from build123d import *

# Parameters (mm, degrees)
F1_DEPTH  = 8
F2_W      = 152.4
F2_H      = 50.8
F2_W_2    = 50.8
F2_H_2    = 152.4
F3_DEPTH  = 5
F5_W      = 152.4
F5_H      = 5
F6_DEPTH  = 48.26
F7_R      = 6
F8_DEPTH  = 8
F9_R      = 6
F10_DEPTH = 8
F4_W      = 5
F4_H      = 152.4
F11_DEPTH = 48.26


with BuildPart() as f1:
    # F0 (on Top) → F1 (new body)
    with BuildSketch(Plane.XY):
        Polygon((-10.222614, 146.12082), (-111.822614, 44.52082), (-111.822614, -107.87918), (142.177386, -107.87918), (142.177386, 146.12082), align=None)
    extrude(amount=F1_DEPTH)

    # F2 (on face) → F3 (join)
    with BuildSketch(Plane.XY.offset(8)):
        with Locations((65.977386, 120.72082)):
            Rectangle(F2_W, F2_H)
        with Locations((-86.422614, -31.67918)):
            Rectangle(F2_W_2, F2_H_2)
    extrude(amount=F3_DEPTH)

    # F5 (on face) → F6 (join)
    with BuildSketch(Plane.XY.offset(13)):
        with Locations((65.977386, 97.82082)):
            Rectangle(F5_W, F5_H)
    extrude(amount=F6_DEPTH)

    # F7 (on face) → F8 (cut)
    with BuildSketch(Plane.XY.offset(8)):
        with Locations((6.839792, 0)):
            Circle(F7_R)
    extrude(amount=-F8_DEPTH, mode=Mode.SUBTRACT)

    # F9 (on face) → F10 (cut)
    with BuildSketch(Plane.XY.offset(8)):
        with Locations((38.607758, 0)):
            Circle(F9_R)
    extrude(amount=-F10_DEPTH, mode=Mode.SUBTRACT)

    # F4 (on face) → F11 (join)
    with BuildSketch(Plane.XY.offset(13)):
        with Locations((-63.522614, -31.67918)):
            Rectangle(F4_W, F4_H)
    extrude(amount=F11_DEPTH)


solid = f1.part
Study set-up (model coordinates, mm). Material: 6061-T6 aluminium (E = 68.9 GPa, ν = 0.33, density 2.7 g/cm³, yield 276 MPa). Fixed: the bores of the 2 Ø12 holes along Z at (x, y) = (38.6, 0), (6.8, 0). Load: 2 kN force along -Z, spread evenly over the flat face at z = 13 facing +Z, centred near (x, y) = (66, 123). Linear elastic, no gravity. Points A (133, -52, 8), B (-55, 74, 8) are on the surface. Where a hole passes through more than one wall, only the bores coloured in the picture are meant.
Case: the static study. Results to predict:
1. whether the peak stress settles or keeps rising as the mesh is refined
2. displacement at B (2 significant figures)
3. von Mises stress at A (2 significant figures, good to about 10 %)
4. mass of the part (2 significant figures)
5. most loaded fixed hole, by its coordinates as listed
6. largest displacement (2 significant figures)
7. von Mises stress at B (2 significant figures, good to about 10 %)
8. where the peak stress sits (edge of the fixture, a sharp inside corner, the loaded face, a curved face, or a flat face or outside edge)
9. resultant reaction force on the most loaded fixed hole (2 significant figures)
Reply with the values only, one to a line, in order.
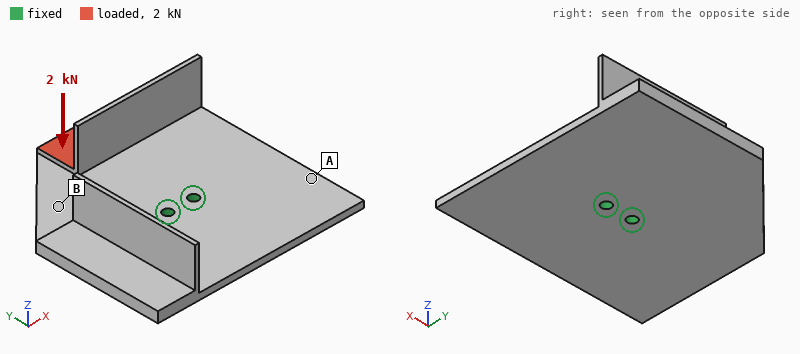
keeps rising
0.58 mm
19 MPa
1.7 kg
(38.6, 0)
3.8 mm
56 MPa
edge of the fixture
2.4 kN
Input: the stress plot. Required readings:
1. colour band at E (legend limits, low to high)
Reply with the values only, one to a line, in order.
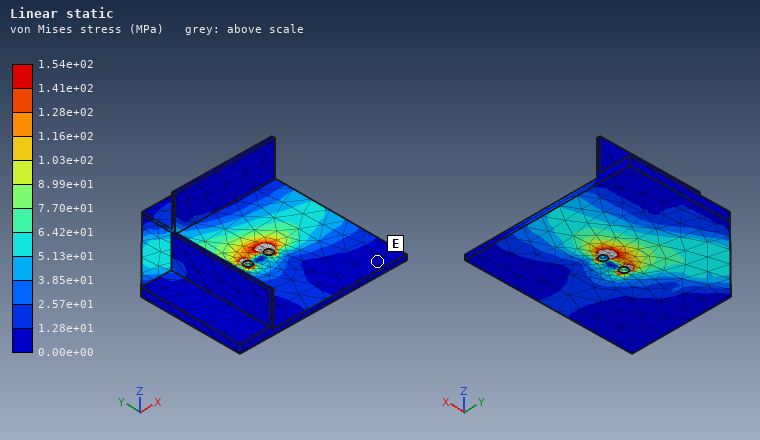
0.00e+00 to 1.28e+01 MPa
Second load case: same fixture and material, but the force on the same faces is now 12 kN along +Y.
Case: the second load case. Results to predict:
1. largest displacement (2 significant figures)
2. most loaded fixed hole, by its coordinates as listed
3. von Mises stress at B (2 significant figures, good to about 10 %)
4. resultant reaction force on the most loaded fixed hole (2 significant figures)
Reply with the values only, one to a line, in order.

2.0 mm
(38.6, 0)
38 MPa
19 kN
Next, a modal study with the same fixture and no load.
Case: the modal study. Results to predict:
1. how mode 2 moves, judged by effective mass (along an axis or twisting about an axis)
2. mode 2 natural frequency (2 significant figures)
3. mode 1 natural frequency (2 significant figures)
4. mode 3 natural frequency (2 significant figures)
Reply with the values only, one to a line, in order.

along Z
310 Hz
210 Hz
390 Hz
